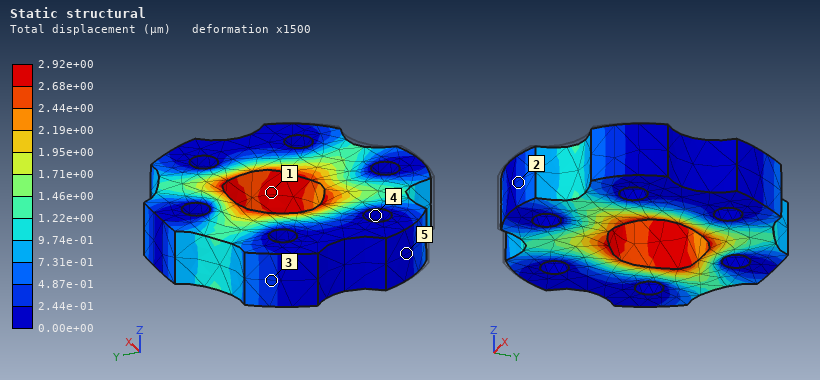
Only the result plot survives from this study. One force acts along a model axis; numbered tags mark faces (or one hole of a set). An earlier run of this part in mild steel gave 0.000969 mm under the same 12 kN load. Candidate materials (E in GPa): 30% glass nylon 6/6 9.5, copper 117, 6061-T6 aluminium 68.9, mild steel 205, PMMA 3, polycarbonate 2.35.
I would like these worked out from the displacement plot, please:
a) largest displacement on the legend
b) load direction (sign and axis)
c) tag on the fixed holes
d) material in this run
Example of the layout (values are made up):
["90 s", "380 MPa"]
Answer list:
["2.92e+00 µm", "+Y", "4", "6061-T6 aluminium"]
